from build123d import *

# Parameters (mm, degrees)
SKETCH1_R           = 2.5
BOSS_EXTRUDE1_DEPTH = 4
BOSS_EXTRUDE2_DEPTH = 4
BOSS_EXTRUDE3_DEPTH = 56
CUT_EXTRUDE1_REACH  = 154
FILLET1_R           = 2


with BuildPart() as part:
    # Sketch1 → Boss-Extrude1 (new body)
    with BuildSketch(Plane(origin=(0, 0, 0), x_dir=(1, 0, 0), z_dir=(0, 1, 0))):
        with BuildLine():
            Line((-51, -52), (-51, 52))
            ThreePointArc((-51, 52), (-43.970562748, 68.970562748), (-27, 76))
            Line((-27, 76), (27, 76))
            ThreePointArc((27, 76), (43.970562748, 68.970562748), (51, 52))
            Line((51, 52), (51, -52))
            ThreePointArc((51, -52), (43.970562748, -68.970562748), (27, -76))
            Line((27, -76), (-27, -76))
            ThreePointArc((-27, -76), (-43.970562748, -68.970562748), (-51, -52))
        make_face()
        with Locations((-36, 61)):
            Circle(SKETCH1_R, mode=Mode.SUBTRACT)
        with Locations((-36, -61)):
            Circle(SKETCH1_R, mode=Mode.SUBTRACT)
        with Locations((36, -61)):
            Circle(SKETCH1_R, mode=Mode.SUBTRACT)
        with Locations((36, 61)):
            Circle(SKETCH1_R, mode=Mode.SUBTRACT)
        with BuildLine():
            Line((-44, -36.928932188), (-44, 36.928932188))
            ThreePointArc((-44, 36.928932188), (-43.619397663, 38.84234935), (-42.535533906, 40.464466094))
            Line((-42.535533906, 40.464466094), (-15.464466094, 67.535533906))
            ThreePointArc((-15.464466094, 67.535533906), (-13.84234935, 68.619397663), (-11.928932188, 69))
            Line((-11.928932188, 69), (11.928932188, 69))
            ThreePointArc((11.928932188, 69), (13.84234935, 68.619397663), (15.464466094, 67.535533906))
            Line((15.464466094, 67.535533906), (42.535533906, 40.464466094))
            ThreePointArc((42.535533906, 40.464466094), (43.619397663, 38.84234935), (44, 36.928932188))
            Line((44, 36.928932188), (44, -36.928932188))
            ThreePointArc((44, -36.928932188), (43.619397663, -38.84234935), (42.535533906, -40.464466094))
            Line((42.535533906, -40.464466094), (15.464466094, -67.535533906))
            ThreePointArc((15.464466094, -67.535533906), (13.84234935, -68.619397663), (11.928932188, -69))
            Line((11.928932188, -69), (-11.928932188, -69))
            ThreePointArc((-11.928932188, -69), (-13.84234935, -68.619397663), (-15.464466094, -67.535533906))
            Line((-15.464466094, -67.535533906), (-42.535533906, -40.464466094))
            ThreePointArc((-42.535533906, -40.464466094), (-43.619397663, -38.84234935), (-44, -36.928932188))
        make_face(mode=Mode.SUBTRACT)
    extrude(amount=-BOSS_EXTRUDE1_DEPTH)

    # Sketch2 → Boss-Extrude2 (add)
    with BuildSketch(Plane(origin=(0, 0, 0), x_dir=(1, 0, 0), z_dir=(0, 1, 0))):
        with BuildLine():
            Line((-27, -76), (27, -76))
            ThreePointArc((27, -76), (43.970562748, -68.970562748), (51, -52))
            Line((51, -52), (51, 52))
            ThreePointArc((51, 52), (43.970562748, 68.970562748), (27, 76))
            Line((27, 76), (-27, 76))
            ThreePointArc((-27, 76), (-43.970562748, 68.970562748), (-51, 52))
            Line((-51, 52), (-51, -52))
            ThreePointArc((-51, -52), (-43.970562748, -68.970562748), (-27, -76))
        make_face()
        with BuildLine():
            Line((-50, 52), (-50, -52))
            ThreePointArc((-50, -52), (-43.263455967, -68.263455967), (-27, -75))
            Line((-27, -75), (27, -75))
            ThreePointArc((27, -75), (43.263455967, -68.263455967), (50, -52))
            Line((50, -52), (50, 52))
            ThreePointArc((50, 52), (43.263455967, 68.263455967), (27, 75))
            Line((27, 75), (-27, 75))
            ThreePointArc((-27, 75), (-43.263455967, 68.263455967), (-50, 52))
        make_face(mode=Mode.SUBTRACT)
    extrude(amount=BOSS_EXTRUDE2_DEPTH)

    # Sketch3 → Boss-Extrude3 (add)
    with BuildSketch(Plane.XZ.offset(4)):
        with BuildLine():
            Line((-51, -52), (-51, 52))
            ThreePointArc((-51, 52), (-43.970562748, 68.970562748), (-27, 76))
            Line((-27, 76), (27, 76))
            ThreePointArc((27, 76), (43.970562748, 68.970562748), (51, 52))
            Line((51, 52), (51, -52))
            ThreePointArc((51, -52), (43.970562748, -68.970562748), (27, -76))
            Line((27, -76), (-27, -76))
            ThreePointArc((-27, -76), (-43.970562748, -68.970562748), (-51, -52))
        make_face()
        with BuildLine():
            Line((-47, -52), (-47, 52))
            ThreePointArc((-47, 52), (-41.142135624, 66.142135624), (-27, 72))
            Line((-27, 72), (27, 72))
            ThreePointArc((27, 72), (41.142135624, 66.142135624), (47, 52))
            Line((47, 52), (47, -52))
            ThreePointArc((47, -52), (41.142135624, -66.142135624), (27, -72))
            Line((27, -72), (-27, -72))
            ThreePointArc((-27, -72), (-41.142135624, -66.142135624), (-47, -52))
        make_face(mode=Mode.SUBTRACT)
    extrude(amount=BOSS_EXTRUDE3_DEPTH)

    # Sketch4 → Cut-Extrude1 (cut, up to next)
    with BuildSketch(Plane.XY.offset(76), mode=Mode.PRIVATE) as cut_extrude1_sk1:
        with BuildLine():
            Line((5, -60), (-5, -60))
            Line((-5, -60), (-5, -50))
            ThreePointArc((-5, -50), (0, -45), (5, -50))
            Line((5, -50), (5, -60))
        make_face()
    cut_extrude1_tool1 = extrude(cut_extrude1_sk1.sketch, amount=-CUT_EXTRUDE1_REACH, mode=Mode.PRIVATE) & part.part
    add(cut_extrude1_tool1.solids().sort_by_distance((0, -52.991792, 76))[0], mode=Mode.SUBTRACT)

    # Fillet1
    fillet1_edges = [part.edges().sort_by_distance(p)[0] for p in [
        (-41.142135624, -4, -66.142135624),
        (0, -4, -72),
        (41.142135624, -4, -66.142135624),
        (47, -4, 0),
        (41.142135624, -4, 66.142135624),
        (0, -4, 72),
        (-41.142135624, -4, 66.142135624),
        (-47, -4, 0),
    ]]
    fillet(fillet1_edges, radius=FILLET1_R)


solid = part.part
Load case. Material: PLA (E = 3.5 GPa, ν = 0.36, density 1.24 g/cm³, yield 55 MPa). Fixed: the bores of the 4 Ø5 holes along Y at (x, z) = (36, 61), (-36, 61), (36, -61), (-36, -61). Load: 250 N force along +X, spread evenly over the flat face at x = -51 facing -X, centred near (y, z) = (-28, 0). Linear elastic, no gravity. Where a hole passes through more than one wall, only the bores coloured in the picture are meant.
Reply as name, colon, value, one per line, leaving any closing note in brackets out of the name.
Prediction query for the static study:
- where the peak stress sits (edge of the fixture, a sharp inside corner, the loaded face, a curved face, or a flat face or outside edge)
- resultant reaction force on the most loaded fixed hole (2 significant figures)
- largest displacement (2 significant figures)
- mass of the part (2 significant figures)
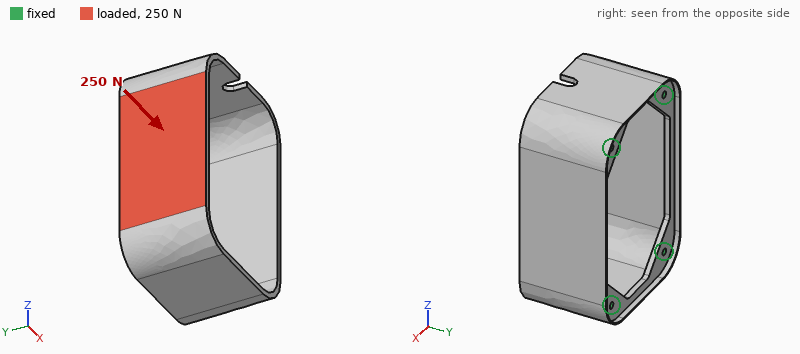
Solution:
where the peak stress sits: a curved face
resultant reaction force on the most loaded fixed hole: 190 N
largest displacement: 2.3 mm
mass of the part: 150 g
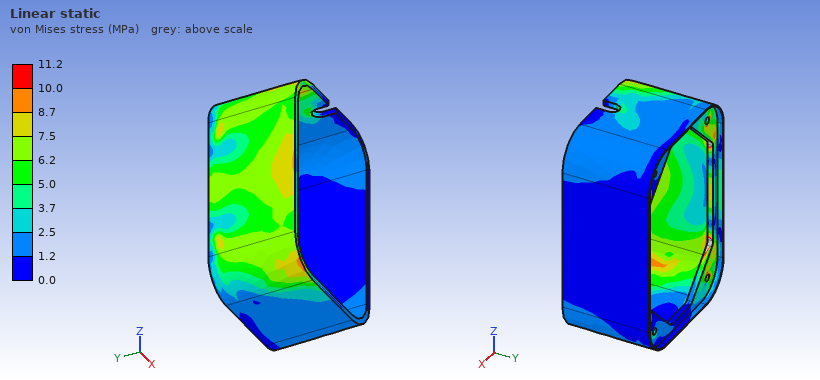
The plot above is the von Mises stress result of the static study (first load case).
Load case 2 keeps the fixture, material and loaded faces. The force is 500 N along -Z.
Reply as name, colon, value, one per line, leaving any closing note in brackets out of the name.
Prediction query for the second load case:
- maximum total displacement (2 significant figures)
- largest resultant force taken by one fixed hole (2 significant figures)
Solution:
maximum total displacement: 0.15 mm
largest resultant force taken by one fixed hole: 280 N
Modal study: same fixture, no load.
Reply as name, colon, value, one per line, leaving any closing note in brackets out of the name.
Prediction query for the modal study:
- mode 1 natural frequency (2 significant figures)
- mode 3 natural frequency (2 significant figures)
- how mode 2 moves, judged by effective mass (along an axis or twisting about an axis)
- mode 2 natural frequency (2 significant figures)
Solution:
mode 1 natural frequency: 330 Hz
mode 3 natural frequency: 640 Hz
how mode 2 moves, judged by effective mass: along X
mode 2 natural frequency: 410 Hz
